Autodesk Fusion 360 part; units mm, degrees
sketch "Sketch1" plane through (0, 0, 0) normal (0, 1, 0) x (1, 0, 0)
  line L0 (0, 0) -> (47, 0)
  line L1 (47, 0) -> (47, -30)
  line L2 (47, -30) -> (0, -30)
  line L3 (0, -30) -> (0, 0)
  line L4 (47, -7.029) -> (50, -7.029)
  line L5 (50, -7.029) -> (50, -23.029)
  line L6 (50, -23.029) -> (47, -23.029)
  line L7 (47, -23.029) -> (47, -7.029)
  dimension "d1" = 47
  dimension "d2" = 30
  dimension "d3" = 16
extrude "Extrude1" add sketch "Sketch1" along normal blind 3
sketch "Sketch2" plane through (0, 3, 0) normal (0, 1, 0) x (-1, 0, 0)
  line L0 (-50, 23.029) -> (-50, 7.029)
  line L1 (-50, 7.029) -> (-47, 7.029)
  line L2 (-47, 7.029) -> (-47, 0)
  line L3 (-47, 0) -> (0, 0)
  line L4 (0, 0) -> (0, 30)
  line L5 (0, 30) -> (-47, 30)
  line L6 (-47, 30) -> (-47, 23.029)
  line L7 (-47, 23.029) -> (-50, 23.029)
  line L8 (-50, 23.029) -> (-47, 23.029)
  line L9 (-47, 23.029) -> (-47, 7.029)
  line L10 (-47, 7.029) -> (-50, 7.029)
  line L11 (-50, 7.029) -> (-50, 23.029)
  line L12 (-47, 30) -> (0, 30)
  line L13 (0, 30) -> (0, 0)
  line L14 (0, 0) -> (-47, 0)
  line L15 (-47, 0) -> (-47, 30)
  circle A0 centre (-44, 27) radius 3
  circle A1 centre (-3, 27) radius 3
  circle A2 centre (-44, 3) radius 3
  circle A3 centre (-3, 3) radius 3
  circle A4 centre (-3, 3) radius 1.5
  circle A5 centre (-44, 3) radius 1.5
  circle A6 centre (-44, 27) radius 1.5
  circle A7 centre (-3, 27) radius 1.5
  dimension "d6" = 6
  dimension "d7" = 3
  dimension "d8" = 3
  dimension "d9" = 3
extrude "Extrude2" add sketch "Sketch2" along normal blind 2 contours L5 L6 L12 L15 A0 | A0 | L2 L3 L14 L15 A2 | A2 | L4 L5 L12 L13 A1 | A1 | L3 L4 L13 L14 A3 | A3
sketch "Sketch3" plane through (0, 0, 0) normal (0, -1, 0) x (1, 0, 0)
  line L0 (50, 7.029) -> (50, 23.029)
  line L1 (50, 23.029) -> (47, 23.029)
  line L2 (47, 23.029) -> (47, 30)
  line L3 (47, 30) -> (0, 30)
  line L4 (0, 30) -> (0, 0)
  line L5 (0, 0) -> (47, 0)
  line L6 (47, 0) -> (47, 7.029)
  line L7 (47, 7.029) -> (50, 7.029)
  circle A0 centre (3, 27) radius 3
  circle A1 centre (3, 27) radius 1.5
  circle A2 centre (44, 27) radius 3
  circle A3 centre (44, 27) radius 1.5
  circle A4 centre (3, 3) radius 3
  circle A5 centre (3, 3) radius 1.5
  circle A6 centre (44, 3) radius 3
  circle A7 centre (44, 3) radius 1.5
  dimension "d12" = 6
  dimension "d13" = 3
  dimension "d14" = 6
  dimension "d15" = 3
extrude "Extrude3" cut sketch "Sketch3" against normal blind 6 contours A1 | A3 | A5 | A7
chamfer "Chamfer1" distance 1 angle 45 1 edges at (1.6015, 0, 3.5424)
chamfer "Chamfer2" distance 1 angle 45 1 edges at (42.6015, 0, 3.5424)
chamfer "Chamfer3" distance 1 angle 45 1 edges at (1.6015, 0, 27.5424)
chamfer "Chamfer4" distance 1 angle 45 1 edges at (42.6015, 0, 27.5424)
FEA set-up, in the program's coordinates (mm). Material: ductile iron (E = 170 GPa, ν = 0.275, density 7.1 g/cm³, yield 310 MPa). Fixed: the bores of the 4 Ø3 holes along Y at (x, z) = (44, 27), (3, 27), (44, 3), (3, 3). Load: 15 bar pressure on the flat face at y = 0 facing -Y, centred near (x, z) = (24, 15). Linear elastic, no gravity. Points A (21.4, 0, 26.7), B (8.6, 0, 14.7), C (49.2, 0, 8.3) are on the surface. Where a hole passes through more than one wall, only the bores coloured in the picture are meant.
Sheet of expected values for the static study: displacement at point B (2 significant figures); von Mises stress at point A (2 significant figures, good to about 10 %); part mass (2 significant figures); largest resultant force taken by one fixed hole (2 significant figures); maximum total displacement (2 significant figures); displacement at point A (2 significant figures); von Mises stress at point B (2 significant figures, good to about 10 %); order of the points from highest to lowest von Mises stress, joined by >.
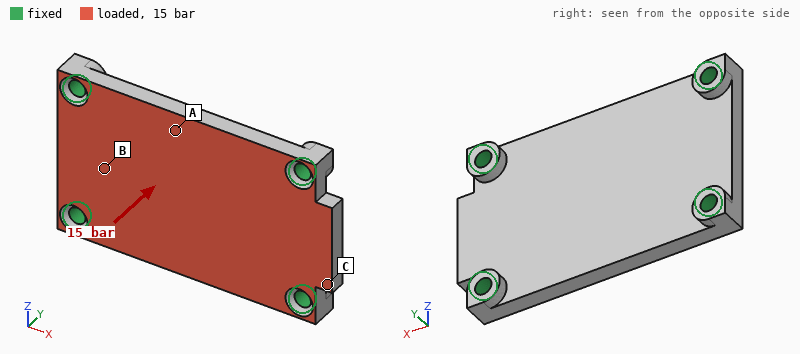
15 µm
78 MPa
32 g
600 N
36 µm
33 µm
38 MPa
A > B > C
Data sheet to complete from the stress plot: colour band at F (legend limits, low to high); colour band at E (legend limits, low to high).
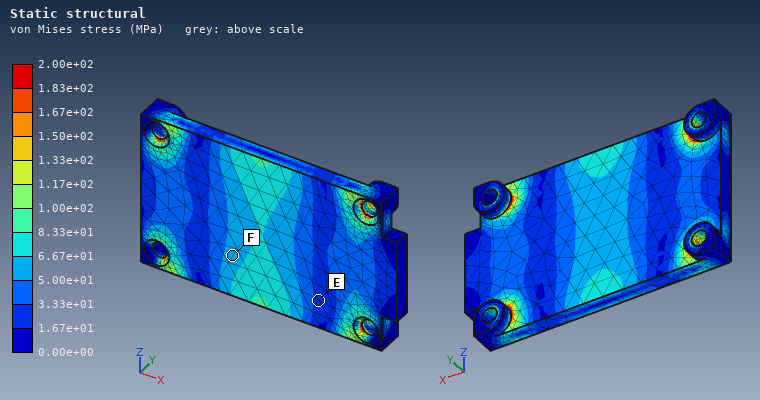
5.00e+01 to 6.67e+01 MPa
1.67e+01 to 3.33e+01 MPa
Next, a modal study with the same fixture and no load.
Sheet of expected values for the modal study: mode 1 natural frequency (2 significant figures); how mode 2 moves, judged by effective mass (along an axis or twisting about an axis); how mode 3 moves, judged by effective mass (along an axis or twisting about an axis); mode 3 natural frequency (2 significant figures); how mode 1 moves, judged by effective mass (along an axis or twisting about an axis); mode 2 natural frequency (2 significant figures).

8000 Hz
twisting about X
twisting about Z
20 kHz
along Y
12 kHz
